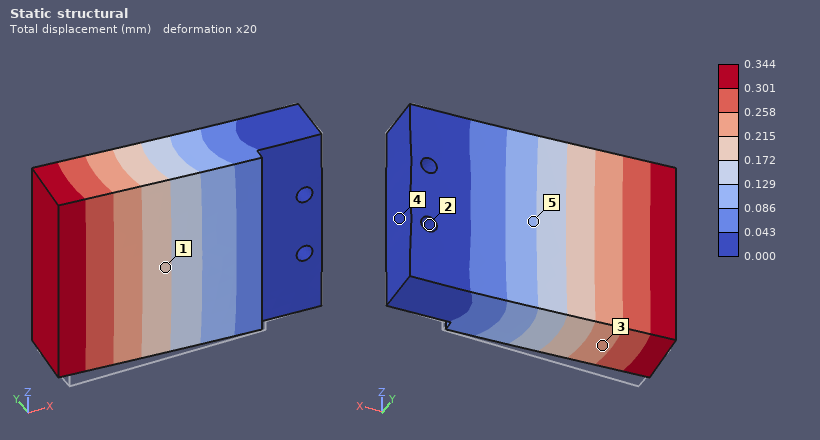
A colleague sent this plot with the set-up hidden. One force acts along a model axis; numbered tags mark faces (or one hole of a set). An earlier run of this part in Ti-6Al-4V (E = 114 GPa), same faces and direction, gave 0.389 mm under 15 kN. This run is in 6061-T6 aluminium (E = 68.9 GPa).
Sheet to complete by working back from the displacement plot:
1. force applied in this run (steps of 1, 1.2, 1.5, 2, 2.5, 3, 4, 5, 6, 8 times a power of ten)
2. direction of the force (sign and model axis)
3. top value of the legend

8 kN
+Y
0.344 mm
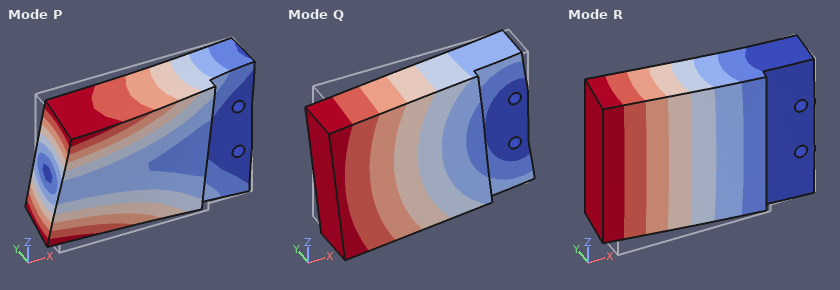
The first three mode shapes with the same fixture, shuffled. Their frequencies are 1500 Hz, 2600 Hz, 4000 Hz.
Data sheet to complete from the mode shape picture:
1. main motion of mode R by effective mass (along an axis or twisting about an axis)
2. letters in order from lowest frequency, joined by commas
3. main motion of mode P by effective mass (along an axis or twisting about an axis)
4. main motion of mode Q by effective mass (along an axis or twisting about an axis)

along Y
R, Q, P
twisting about X
along Z
